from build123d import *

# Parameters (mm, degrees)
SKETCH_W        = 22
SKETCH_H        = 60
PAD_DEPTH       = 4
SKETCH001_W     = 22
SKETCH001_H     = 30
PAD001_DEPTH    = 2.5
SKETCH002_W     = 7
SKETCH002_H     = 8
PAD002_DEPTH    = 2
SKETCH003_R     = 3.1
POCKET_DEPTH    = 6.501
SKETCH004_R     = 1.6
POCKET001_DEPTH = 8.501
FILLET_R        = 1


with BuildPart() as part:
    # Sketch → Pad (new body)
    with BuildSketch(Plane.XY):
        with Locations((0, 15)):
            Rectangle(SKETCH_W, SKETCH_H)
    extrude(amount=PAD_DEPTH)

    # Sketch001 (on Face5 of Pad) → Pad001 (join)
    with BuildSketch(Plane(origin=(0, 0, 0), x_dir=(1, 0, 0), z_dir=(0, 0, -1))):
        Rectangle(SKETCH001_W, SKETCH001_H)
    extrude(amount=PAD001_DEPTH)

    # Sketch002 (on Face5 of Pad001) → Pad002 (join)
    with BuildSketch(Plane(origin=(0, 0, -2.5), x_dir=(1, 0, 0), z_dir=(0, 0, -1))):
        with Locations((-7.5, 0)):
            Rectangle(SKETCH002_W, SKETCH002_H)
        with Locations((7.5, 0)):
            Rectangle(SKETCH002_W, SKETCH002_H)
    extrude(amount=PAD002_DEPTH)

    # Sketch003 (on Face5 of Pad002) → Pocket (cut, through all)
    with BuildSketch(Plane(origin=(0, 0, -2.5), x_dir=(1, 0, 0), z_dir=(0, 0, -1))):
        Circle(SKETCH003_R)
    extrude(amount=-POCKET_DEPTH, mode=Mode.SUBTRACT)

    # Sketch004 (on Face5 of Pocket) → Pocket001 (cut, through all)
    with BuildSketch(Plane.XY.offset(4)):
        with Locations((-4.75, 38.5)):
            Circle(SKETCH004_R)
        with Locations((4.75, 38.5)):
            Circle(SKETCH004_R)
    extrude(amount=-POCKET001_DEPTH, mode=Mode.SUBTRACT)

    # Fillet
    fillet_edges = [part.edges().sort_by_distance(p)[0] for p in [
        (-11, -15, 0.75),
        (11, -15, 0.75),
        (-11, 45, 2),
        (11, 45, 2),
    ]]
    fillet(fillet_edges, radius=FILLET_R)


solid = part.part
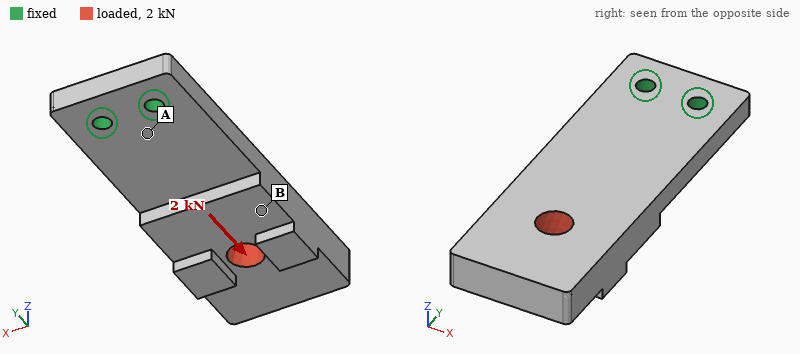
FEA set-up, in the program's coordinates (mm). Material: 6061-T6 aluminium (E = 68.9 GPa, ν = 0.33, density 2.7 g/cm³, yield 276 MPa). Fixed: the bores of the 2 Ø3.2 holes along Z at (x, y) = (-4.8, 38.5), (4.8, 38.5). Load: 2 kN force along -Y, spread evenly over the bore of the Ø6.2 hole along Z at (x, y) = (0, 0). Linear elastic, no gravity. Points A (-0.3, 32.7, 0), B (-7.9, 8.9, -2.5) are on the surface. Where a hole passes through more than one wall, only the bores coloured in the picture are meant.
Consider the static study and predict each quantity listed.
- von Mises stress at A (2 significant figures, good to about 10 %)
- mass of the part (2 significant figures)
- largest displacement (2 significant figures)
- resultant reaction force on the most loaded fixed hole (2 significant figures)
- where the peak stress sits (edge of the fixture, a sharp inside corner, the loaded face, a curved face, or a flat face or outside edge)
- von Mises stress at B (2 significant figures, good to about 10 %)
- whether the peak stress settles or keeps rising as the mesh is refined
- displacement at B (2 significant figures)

61 MPa
19 g
0.30 mm
1.0 kN
edge of the fixture
14 MPa
keeps rising
0.13 mm
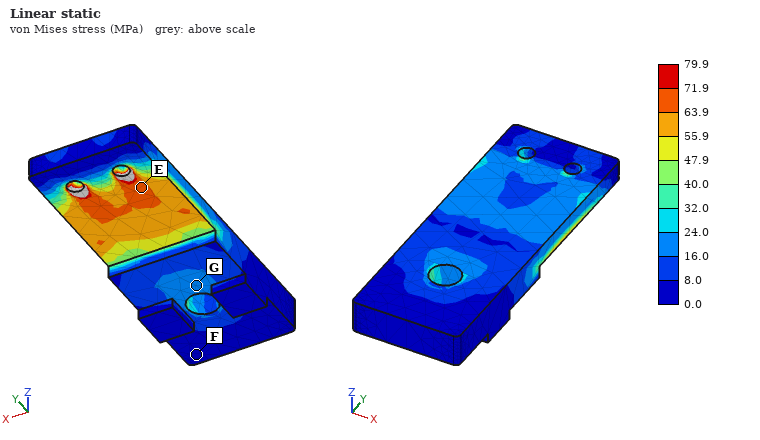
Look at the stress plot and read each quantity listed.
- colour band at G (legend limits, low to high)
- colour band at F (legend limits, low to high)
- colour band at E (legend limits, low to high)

16.0 to 24.0 MPa
0.0 to 8.0 MPa
63.9 to 71.9 MPa
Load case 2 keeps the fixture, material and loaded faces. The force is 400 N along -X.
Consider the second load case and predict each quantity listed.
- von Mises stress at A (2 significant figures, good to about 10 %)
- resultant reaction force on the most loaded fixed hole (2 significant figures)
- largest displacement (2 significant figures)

27 MPa
1.3 kN
73 µm
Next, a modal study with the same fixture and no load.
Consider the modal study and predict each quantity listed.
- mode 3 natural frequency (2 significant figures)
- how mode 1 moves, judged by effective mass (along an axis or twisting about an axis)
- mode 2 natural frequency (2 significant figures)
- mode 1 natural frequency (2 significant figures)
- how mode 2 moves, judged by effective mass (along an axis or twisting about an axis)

4800 Hz
along Z
3900 Hz
950 Hz
along X
